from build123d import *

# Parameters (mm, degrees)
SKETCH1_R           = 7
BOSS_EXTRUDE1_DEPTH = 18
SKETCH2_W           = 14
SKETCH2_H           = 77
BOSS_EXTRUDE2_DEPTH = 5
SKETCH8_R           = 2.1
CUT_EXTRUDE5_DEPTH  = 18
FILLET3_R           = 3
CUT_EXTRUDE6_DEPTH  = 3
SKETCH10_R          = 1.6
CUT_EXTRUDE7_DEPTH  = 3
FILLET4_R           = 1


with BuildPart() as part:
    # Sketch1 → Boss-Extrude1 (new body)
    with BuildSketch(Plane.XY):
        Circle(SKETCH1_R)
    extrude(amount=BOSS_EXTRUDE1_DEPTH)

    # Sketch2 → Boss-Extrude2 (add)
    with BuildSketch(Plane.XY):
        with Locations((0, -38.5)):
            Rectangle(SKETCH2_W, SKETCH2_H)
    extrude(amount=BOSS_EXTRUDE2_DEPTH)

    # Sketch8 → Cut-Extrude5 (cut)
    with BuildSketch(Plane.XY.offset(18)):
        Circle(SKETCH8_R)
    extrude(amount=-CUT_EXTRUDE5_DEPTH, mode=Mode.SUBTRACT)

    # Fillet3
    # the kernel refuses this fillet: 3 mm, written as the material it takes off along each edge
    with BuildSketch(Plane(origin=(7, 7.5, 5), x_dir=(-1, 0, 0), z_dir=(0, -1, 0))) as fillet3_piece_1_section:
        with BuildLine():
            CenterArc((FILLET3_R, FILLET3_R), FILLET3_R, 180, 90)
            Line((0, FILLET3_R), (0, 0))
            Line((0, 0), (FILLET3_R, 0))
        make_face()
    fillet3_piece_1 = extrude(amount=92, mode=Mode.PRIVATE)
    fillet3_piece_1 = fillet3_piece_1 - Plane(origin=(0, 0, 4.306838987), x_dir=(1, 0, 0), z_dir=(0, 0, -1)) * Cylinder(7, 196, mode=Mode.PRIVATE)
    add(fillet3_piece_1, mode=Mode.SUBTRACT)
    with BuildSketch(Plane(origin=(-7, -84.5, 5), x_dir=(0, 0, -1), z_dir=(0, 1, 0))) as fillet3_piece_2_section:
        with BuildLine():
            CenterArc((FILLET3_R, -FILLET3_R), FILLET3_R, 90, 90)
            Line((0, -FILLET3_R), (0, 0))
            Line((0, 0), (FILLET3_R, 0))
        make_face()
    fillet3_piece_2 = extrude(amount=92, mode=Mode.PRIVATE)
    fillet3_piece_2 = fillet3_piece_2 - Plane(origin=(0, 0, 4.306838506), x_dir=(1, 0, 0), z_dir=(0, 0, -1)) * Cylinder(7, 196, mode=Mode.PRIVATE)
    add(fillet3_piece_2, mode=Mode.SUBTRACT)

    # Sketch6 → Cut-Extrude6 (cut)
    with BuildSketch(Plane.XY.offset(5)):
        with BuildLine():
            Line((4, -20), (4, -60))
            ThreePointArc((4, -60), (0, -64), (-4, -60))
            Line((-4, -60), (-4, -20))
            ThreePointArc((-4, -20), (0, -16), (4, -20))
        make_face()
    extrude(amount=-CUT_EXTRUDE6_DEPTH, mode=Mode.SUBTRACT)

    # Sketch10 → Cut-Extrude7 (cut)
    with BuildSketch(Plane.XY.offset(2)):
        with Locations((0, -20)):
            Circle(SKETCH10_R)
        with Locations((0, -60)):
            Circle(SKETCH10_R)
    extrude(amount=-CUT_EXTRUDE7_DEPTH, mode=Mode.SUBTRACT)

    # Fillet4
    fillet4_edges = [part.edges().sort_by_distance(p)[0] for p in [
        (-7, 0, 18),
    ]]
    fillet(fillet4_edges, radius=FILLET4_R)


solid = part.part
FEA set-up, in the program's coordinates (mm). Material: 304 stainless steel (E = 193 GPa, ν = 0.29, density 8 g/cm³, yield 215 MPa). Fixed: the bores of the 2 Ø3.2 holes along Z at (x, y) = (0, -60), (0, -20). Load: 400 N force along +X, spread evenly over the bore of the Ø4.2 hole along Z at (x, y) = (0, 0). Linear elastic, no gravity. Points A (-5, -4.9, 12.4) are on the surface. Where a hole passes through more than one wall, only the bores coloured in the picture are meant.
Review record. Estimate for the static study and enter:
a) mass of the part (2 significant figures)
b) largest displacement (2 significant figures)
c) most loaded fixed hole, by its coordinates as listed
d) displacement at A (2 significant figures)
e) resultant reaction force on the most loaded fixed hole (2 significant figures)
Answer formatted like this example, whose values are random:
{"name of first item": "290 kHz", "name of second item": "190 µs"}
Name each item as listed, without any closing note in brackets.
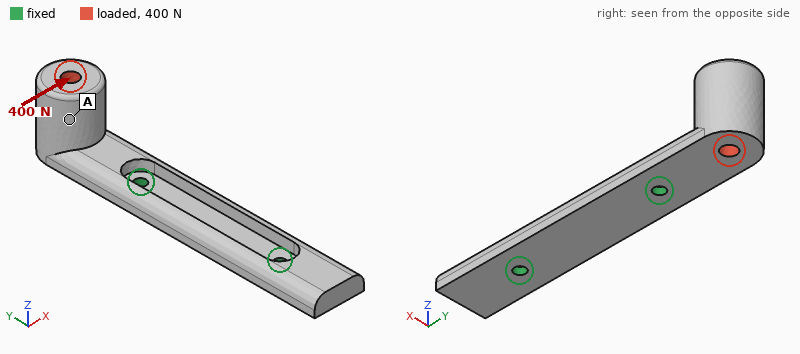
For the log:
{"mass of the part": "49 g", "largest displacement": "68 µm", "most loaded fixed hole, by its coordinates as listed": "(0, -20)", "displacement at A": "46 µm", "resultant reaction force on the most loaded fixed hole": "540 N"}
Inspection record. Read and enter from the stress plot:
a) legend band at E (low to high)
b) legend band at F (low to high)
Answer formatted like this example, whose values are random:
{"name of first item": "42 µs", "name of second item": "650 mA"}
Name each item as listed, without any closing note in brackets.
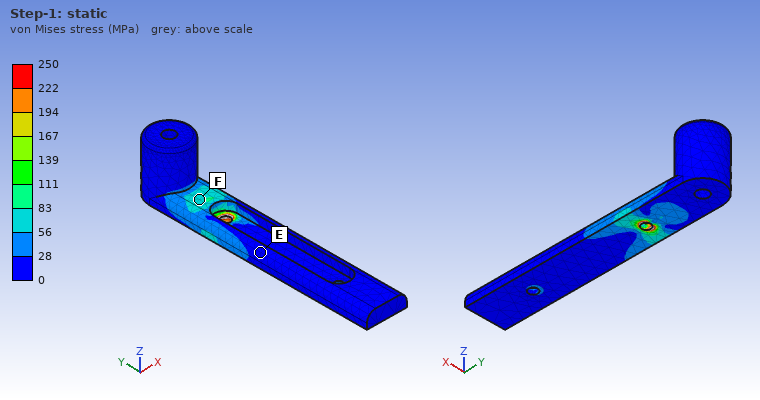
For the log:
{"legend band at E": "0 to 28 MPa", "legend band at F": "56 to 83 MPa"}
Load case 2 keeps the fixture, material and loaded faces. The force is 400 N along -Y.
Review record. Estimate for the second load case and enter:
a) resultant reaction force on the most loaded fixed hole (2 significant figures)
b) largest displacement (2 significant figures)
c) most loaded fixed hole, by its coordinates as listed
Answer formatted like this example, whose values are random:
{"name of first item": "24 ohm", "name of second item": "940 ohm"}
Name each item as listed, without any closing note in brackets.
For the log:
{"resultant reaction force on the most loaded fixed hole": "220 N", "largest displacement": "84 µm", "most loaded fixed hole, by its coordinates as listed": "(0, -60)"}
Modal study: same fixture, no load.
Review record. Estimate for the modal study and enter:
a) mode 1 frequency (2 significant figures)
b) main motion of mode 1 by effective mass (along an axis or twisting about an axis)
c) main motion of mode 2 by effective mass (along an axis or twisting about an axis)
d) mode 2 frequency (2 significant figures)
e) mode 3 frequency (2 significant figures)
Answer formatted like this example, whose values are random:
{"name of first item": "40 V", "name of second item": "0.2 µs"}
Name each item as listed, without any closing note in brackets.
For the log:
{"mode 1 frequency": "1900 Hz", "main motion of mode 1 by effective mass": "along Z", "main motion of mode 2 by effective mass": "along X", "mode 2 frequency": "3200 Hz", "mode 3 frequency": "6900 Hz"}
